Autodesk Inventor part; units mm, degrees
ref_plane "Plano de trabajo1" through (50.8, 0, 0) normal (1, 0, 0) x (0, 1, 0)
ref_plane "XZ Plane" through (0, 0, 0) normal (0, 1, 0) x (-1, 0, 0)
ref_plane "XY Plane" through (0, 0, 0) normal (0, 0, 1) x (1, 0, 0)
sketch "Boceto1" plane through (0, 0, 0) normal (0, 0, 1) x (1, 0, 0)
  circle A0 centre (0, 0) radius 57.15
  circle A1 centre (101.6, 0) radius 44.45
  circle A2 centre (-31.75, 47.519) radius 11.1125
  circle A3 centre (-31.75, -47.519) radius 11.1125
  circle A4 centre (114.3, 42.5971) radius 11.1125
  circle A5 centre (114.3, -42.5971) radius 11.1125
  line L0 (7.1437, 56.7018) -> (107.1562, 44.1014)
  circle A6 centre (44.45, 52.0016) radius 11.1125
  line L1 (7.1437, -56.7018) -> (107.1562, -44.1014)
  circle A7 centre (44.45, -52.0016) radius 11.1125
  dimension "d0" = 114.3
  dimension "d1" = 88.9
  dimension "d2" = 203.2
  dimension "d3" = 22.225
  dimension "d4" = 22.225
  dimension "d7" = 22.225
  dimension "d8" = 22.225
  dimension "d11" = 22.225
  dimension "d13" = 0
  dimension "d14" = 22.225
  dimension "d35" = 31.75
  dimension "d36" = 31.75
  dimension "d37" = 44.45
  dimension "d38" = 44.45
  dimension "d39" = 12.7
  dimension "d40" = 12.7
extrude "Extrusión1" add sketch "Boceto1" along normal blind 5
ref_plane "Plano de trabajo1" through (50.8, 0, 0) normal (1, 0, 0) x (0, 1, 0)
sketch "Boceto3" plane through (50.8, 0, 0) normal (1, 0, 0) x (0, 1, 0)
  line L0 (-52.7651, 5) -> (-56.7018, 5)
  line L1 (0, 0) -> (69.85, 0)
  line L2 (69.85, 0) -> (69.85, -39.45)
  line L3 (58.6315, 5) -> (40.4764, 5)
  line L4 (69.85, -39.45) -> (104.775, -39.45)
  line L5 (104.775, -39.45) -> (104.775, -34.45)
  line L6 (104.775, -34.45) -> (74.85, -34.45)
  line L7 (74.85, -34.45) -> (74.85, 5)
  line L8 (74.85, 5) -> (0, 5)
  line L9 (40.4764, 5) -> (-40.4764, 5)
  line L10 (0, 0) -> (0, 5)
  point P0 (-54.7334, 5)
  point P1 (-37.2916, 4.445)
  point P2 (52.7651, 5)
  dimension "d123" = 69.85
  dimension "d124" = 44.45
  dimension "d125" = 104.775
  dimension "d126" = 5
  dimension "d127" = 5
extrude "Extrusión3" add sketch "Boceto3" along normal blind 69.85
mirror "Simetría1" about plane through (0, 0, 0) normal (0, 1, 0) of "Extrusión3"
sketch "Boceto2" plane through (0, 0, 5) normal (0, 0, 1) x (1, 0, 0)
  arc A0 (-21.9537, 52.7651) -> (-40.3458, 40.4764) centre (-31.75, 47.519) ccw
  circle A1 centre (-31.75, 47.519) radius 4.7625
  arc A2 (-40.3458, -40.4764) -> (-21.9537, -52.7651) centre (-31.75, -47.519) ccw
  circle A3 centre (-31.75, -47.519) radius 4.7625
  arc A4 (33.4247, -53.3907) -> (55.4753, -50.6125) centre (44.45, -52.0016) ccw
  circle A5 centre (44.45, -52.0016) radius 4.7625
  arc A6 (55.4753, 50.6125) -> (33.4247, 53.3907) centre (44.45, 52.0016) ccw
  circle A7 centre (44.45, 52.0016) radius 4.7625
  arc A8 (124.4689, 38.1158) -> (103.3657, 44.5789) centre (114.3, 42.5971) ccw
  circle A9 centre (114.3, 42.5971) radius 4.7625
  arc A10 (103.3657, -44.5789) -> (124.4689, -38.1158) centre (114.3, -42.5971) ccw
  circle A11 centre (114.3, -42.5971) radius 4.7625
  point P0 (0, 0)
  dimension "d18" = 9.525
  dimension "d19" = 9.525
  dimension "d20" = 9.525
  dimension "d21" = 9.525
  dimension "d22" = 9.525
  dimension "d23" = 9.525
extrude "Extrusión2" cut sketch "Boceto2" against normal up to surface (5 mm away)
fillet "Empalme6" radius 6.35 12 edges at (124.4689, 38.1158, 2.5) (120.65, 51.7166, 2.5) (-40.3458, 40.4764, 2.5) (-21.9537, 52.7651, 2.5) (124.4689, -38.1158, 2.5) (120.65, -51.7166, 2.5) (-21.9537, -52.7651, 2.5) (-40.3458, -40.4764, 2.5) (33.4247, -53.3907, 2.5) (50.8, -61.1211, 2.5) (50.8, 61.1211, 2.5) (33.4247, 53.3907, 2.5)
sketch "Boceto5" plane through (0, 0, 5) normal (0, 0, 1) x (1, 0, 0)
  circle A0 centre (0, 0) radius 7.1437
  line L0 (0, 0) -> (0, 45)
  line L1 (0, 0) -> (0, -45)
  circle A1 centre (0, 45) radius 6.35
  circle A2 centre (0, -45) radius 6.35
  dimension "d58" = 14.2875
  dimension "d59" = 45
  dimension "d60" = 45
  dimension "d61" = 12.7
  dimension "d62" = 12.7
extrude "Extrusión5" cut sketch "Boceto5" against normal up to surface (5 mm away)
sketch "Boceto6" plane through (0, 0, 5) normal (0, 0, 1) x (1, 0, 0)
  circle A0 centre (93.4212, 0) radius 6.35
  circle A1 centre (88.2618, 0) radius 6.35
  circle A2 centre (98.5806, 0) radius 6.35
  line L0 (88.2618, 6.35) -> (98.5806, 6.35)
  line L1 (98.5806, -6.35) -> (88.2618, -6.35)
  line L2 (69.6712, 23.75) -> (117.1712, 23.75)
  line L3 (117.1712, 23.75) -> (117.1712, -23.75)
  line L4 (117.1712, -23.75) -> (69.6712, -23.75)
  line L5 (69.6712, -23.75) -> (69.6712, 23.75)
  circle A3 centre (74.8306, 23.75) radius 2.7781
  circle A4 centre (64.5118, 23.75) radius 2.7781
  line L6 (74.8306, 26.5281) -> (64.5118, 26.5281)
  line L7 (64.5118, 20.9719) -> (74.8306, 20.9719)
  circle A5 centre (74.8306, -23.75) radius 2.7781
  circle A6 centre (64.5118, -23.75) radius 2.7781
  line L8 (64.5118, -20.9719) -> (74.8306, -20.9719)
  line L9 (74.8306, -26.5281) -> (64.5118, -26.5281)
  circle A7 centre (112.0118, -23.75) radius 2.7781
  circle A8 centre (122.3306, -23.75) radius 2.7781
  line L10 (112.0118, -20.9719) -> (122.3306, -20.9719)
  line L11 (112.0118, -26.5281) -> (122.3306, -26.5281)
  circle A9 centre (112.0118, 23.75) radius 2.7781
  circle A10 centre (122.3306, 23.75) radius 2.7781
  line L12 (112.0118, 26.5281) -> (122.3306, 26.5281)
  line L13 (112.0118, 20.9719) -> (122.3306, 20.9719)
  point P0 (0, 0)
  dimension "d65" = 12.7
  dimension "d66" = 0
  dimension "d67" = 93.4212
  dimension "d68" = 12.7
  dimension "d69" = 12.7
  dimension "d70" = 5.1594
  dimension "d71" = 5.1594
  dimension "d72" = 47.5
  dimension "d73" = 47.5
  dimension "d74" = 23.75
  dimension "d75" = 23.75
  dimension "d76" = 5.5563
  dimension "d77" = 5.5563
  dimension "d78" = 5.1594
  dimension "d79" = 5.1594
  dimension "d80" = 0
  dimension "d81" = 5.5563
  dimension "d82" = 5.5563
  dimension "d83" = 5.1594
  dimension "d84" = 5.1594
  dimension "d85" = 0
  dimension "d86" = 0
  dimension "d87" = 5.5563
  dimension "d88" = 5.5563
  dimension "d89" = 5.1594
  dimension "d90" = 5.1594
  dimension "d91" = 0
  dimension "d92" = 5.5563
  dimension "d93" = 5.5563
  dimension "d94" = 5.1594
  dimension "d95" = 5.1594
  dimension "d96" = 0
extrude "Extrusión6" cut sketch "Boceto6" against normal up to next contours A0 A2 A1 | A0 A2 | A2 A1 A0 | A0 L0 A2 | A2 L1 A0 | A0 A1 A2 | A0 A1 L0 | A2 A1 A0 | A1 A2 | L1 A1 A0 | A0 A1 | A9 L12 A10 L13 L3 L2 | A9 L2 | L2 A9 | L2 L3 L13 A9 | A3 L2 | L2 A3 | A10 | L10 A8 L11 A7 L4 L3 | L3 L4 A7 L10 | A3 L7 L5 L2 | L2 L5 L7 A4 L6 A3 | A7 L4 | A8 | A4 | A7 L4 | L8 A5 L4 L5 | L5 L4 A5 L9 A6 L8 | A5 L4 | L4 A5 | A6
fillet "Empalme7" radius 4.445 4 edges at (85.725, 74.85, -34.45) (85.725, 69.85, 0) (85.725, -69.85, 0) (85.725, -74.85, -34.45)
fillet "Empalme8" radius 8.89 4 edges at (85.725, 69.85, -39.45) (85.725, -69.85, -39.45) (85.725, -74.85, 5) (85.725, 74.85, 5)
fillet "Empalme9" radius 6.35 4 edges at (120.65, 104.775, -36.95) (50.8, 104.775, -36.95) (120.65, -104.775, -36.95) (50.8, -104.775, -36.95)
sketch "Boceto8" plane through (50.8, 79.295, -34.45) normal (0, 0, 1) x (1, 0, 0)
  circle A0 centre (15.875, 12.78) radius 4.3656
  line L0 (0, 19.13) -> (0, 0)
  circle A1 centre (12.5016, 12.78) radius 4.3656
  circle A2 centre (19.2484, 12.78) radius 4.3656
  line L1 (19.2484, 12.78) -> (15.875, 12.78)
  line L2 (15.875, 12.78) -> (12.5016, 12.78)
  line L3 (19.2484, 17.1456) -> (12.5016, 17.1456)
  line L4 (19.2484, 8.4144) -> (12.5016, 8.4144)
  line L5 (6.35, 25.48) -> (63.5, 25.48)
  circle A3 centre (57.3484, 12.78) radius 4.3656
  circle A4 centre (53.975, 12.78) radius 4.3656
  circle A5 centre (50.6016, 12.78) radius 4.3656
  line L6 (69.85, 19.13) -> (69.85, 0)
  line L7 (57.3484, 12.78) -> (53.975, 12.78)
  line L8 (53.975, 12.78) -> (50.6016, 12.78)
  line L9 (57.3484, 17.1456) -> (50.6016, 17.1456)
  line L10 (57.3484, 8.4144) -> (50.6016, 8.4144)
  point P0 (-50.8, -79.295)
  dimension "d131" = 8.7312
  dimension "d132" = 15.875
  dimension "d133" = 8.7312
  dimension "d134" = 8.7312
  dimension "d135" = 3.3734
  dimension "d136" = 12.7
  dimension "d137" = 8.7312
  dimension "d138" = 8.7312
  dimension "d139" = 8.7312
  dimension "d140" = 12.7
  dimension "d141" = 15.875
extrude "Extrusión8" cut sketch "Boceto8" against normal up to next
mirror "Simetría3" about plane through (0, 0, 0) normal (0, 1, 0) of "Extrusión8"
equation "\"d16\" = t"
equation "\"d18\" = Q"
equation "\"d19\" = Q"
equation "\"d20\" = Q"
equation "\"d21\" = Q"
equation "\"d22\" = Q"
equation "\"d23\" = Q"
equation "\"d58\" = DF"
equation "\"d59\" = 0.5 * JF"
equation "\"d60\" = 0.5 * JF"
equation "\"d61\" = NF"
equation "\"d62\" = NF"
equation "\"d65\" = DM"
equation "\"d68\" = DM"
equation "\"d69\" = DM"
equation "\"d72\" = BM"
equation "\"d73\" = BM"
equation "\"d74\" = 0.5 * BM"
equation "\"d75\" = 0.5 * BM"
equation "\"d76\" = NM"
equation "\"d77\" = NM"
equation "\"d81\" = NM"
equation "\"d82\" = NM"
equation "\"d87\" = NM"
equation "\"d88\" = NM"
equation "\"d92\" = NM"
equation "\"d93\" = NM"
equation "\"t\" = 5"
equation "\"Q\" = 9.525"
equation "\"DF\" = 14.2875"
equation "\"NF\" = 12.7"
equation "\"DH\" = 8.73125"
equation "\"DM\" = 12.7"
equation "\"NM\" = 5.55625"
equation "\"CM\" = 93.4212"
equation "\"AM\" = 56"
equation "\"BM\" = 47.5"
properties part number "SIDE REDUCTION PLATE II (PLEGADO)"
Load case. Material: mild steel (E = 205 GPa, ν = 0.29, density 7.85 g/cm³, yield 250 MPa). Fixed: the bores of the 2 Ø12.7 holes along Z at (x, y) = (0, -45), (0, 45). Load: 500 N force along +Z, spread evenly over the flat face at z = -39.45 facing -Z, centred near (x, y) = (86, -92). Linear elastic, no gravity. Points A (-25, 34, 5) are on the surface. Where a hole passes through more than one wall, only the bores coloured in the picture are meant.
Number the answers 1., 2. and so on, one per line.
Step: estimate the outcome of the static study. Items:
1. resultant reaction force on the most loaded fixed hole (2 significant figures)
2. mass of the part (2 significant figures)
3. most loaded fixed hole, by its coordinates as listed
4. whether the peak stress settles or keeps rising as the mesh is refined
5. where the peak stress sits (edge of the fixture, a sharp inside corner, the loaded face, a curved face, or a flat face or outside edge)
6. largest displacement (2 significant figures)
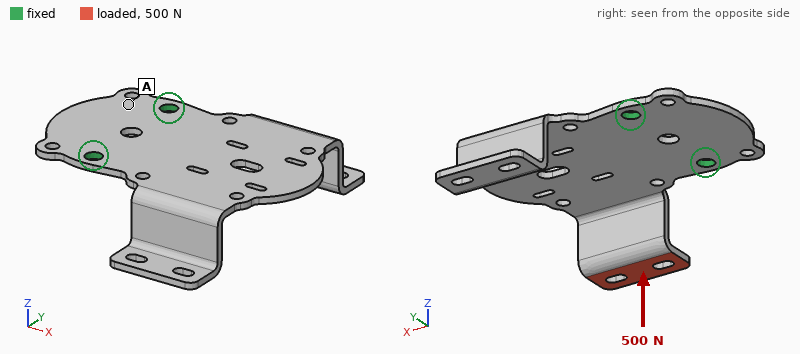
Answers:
1. 730 N
2. 1.2 kg
3. (0, -45)
4. keeps rising
5. edge of the fixture
6. 1.8 mm
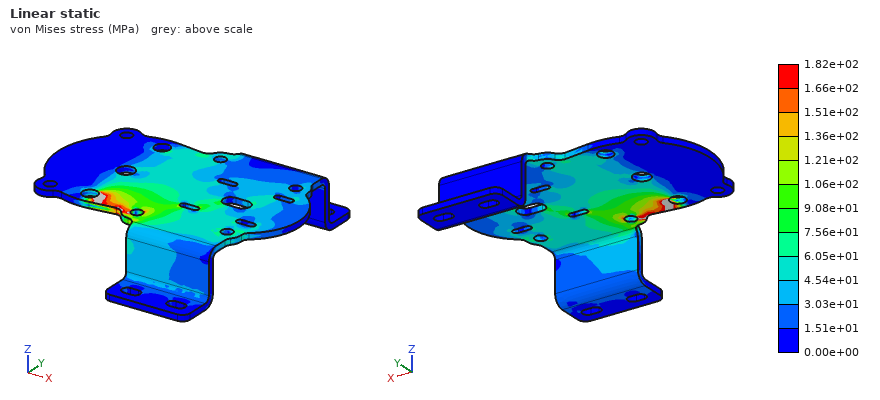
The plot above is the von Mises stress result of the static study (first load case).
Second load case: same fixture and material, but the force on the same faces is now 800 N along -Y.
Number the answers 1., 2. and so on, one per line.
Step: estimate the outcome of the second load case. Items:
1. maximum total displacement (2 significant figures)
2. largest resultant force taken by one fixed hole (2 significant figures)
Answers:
1. 1.2 mm
2. 900 N
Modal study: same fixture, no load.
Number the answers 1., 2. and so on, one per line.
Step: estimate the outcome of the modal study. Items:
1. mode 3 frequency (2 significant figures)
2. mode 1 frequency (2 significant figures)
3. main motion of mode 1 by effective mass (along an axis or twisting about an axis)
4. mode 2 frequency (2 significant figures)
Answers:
1. 450 Hz
2. 160 Hz
3. along Z
4. 250 Hz
